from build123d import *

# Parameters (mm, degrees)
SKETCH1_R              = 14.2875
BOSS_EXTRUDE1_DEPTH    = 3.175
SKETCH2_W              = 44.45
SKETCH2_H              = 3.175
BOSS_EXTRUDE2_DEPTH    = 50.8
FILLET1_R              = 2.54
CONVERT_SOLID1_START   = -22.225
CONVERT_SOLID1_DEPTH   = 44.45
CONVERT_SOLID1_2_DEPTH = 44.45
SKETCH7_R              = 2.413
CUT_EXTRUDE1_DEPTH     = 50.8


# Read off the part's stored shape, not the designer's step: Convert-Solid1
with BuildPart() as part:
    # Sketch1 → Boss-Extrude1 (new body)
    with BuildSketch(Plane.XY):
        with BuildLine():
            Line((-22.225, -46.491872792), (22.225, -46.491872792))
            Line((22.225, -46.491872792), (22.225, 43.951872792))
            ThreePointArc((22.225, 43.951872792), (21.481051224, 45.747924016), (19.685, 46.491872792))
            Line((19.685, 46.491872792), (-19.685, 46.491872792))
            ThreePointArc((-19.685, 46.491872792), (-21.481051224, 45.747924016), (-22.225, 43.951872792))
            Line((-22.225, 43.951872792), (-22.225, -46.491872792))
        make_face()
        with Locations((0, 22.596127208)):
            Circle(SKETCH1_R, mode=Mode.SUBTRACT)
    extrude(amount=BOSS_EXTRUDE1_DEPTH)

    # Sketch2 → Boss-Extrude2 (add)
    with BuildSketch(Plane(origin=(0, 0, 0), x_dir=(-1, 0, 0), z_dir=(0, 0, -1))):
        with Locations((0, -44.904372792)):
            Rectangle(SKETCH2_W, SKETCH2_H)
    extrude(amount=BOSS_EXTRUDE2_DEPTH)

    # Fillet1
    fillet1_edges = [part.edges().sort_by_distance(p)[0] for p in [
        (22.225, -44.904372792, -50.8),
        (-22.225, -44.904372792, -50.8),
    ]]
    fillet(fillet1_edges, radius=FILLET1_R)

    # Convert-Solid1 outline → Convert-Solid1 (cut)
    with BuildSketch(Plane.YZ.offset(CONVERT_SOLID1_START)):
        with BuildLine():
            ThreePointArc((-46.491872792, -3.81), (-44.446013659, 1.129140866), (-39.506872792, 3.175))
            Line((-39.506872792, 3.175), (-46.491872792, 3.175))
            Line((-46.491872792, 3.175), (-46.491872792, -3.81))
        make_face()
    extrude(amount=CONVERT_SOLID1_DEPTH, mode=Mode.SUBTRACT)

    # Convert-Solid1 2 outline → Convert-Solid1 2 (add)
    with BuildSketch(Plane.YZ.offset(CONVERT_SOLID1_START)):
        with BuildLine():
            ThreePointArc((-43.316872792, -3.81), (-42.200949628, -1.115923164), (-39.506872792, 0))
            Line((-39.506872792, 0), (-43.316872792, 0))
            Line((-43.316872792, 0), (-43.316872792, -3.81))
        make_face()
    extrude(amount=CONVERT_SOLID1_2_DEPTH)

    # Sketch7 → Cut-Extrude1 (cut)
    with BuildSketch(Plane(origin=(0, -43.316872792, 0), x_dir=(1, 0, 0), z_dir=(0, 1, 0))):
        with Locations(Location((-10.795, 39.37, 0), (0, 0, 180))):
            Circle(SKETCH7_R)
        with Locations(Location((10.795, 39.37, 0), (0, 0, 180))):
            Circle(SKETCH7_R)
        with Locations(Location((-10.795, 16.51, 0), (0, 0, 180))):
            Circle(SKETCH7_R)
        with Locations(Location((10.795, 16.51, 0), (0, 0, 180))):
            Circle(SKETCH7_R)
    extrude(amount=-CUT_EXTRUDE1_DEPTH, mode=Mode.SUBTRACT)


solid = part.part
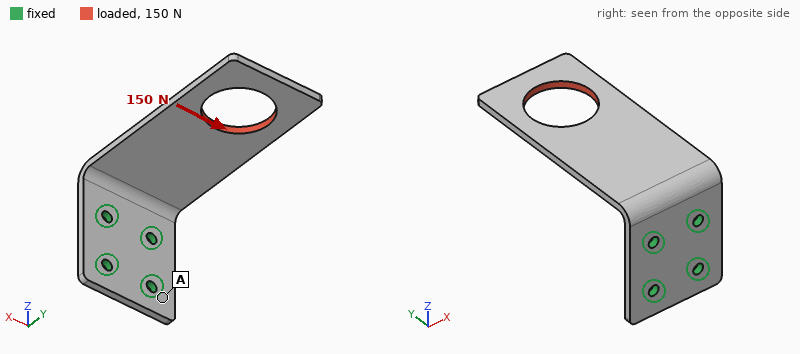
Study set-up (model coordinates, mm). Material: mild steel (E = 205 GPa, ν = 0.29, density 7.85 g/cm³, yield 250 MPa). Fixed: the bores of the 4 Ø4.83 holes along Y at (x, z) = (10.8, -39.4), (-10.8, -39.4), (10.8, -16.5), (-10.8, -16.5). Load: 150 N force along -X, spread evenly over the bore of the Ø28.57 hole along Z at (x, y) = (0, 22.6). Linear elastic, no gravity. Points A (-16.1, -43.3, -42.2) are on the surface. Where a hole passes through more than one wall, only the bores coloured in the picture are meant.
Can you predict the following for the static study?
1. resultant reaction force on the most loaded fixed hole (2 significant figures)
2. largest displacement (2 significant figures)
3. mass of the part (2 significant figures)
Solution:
410 N
0.17 mm
140 g
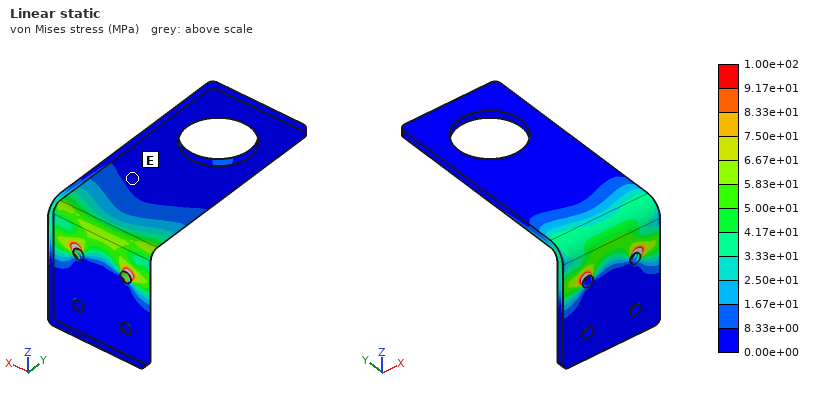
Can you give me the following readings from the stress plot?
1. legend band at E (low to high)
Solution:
0.00e+00 to 8.33e+00 MPa
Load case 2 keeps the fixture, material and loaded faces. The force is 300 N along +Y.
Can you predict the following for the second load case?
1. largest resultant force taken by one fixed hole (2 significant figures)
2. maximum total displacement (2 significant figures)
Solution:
170 N
0.17 mm
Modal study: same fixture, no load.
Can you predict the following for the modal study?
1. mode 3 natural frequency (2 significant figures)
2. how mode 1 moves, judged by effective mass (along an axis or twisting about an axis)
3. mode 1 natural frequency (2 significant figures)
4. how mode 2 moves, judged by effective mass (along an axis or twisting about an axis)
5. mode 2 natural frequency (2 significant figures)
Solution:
1300 Hz
along Z
290 Hz
along X
780 Hz
